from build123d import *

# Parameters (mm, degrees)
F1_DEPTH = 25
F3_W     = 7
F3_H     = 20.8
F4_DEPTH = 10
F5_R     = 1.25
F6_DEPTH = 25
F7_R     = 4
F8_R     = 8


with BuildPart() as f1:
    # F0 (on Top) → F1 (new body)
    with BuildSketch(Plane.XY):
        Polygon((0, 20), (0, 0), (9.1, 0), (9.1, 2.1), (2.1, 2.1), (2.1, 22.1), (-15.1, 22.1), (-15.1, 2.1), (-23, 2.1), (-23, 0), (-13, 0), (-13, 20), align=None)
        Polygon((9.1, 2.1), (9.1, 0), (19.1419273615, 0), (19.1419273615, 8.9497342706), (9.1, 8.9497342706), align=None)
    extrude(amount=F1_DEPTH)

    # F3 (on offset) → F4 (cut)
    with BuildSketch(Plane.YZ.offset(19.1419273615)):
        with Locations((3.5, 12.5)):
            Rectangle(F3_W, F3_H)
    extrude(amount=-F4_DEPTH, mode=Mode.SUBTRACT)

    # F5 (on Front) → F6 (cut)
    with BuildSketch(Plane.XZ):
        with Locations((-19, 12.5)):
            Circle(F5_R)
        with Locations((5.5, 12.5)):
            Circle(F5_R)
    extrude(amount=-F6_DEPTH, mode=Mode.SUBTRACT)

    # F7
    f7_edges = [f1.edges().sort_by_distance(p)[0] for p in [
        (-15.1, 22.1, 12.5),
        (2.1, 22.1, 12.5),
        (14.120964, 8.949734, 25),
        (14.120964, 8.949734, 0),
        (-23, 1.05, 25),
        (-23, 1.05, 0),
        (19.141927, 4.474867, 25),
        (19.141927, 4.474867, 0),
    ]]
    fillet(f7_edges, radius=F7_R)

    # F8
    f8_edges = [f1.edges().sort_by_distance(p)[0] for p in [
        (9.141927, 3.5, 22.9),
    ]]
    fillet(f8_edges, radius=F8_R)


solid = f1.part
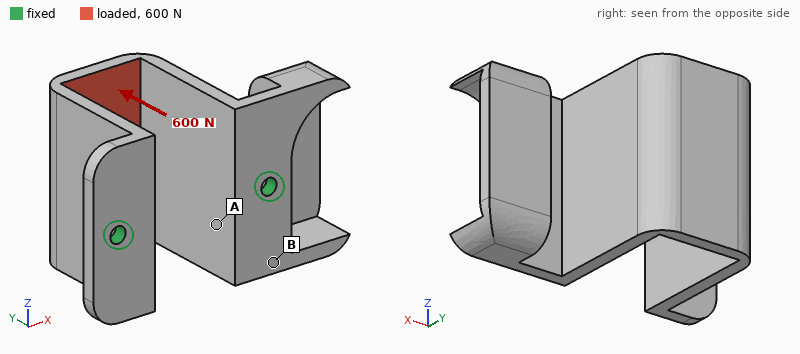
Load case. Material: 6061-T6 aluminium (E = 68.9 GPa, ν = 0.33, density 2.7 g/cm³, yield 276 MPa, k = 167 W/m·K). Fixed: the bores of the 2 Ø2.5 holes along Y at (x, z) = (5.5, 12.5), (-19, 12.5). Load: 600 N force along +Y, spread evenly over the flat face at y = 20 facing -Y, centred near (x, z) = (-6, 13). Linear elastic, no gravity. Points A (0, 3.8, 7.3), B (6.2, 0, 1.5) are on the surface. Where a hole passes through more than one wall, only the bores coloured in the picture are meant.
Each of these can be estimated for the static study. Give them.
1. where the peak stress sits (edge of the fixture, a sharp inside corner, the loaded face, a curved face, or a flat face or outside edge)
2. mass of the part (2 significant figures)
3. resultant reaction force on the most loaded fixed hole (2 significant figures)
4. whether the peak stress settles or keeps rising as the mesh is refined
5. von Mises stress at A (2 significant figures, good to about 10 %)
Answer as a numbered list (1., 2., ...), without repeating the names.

1. edge of the fixture
2. 12 g
3. 310 N
4. keeps rising
5. 15 MPa
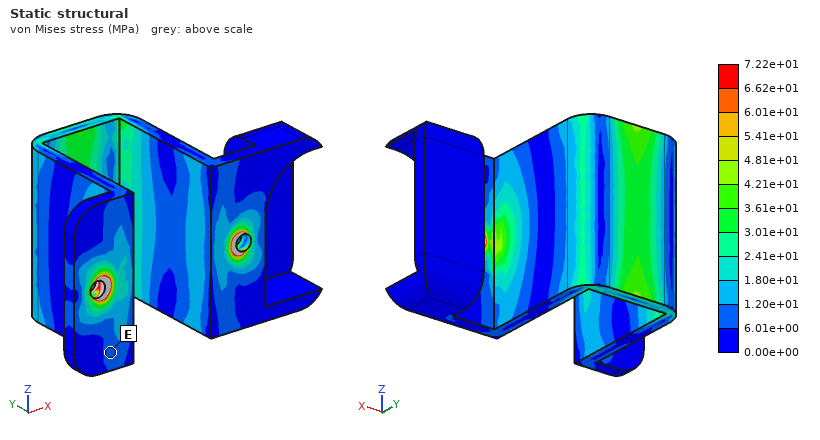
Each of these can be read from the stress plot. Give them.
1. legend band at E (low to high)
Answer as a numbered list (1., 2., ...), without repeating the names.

1. 6.01e+00 to 1.20e+01 MPa
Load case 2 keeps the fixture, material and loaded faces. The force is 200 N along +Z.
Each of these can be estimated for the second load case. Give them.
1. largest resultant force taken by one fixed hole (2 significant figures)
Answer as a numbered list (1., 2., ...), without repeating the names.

1. 100 N
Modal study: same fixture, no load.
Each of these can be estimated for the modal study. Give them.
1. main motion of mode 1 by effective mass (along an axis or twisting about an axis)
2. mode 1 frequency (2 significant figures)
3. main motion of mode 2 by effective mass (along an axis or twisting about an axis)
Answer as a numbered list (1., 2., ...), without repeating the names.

1. along Z
2. 2900 Hz
3. along X
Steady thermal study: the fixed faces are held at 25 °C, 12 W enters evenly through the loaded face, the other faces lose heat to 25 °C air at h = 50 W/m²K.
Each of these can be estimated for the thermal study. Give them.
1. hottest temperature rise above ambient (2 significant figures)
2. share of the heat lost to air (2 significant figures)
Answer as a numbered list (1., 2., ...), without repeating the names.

1. 20 K
2. 16 %
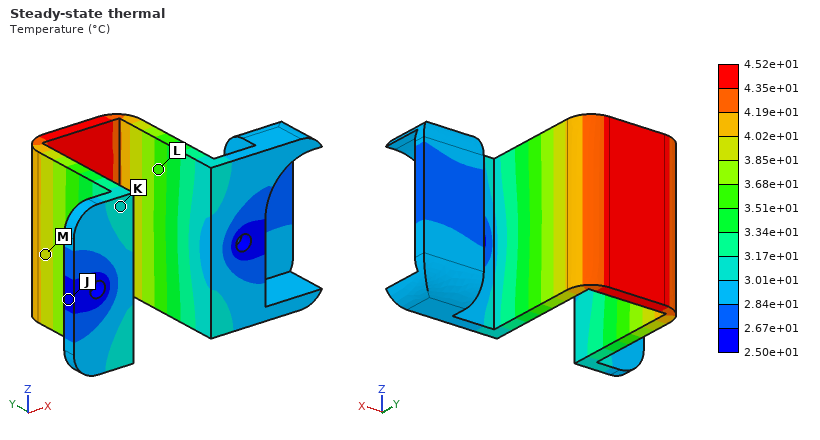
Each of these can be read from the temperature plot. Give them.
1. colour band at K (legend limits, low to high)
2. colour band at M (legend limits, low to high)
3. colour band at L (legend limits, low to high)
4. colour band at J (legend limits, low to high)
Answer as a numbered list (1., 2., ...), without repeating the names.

1. 3.01e+01 to 3.17e+01 °C
2. 3.85e+01 to 4.02e+01 °C
3. 3.51e+01 to 3.68e+01 °C
4. 2.50e+01 to 2.67e+01 °C
